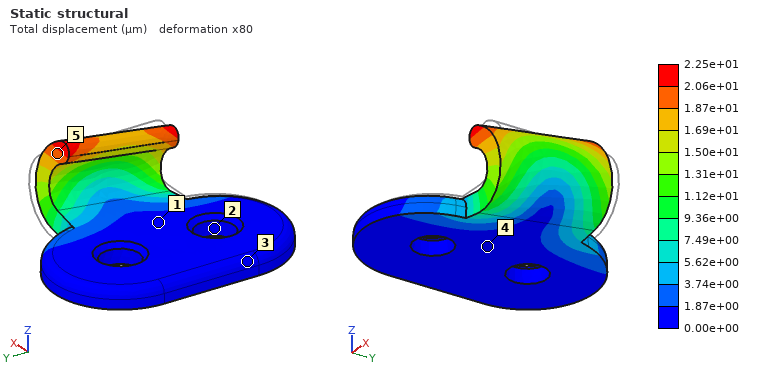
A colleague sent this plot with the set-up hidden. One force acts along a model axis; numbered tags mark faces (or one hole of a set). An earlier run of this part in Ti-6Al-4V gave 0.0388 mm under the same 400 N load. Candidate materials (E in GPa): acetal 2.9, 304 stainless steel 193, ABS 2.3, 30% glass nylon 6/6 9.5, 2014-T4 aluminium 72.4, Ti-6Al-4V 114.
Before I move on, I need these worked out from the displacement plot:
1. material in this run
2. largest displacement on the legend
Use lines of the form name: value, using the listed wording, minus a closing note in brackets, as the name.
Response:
material in this run: 304 stainless steel
largest displacement on the legend: 2.25e+01 µm
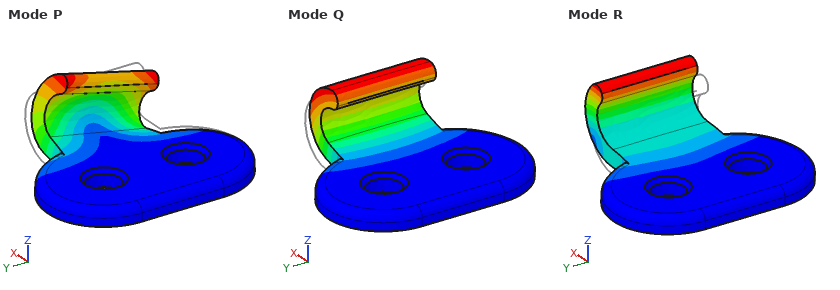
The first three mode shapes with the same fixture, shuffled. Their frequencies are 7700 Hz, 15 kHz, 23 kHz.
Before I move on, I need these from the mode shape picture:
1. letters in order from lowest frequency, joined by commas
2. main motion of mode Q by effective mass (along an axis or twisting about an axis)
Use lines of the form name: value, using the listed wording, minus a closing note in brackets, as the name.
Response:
letters in order from lowest frequency, joined by commas: Q, P, R
main motion of mode Q by effective mass: along Z
